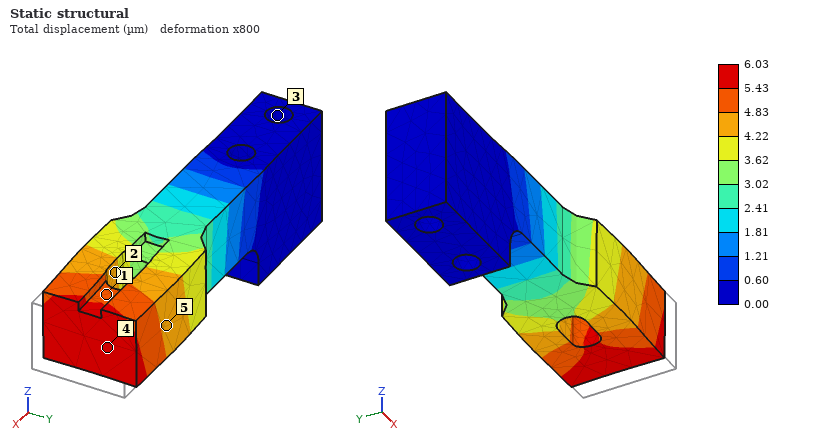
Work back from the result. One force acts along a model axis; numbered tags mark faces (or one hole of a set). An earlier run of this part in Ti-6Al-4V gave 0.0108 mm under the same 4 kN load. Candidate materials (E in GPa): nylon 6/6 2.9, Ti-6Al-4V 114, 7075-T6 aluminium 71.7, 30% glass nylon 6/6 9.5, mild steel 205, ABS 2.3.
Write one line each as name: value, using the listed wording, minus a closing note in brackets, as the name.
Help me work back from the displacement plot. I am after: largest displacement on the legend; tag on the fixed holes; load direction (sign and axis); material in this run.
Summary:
largest displacement on the legend: 6.03 µm
tag on the fixed holes: 3
load direction: -X
material in this run: mild steel
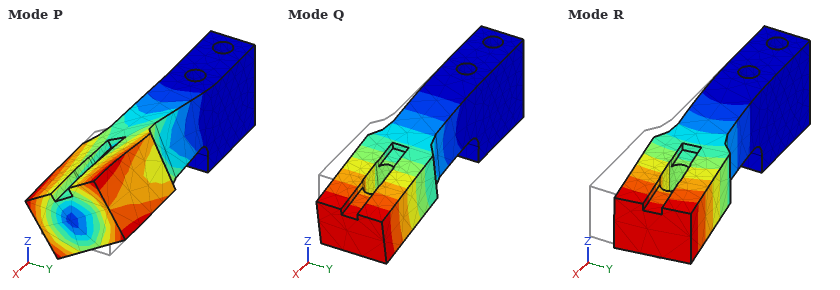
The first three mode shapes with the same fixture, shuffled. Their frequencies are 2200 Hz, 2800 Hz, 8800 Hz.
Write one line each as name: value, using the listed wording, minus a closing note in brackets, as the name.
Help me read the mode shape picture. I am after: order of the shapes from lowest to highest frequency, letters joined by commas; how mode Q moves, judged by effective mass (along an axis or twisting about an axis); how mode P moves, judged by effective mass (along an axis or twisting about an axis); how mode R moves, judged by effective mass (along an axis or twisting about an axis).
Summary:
order of the shapes from lowest to highest frequency, letters joined by commas: R, Q, P
how mode Q moves, judged by effective mass: along Z
how mode P moves, judged by effective mass: twisting about X
how mode R moves, judged by effective mass: along Y
